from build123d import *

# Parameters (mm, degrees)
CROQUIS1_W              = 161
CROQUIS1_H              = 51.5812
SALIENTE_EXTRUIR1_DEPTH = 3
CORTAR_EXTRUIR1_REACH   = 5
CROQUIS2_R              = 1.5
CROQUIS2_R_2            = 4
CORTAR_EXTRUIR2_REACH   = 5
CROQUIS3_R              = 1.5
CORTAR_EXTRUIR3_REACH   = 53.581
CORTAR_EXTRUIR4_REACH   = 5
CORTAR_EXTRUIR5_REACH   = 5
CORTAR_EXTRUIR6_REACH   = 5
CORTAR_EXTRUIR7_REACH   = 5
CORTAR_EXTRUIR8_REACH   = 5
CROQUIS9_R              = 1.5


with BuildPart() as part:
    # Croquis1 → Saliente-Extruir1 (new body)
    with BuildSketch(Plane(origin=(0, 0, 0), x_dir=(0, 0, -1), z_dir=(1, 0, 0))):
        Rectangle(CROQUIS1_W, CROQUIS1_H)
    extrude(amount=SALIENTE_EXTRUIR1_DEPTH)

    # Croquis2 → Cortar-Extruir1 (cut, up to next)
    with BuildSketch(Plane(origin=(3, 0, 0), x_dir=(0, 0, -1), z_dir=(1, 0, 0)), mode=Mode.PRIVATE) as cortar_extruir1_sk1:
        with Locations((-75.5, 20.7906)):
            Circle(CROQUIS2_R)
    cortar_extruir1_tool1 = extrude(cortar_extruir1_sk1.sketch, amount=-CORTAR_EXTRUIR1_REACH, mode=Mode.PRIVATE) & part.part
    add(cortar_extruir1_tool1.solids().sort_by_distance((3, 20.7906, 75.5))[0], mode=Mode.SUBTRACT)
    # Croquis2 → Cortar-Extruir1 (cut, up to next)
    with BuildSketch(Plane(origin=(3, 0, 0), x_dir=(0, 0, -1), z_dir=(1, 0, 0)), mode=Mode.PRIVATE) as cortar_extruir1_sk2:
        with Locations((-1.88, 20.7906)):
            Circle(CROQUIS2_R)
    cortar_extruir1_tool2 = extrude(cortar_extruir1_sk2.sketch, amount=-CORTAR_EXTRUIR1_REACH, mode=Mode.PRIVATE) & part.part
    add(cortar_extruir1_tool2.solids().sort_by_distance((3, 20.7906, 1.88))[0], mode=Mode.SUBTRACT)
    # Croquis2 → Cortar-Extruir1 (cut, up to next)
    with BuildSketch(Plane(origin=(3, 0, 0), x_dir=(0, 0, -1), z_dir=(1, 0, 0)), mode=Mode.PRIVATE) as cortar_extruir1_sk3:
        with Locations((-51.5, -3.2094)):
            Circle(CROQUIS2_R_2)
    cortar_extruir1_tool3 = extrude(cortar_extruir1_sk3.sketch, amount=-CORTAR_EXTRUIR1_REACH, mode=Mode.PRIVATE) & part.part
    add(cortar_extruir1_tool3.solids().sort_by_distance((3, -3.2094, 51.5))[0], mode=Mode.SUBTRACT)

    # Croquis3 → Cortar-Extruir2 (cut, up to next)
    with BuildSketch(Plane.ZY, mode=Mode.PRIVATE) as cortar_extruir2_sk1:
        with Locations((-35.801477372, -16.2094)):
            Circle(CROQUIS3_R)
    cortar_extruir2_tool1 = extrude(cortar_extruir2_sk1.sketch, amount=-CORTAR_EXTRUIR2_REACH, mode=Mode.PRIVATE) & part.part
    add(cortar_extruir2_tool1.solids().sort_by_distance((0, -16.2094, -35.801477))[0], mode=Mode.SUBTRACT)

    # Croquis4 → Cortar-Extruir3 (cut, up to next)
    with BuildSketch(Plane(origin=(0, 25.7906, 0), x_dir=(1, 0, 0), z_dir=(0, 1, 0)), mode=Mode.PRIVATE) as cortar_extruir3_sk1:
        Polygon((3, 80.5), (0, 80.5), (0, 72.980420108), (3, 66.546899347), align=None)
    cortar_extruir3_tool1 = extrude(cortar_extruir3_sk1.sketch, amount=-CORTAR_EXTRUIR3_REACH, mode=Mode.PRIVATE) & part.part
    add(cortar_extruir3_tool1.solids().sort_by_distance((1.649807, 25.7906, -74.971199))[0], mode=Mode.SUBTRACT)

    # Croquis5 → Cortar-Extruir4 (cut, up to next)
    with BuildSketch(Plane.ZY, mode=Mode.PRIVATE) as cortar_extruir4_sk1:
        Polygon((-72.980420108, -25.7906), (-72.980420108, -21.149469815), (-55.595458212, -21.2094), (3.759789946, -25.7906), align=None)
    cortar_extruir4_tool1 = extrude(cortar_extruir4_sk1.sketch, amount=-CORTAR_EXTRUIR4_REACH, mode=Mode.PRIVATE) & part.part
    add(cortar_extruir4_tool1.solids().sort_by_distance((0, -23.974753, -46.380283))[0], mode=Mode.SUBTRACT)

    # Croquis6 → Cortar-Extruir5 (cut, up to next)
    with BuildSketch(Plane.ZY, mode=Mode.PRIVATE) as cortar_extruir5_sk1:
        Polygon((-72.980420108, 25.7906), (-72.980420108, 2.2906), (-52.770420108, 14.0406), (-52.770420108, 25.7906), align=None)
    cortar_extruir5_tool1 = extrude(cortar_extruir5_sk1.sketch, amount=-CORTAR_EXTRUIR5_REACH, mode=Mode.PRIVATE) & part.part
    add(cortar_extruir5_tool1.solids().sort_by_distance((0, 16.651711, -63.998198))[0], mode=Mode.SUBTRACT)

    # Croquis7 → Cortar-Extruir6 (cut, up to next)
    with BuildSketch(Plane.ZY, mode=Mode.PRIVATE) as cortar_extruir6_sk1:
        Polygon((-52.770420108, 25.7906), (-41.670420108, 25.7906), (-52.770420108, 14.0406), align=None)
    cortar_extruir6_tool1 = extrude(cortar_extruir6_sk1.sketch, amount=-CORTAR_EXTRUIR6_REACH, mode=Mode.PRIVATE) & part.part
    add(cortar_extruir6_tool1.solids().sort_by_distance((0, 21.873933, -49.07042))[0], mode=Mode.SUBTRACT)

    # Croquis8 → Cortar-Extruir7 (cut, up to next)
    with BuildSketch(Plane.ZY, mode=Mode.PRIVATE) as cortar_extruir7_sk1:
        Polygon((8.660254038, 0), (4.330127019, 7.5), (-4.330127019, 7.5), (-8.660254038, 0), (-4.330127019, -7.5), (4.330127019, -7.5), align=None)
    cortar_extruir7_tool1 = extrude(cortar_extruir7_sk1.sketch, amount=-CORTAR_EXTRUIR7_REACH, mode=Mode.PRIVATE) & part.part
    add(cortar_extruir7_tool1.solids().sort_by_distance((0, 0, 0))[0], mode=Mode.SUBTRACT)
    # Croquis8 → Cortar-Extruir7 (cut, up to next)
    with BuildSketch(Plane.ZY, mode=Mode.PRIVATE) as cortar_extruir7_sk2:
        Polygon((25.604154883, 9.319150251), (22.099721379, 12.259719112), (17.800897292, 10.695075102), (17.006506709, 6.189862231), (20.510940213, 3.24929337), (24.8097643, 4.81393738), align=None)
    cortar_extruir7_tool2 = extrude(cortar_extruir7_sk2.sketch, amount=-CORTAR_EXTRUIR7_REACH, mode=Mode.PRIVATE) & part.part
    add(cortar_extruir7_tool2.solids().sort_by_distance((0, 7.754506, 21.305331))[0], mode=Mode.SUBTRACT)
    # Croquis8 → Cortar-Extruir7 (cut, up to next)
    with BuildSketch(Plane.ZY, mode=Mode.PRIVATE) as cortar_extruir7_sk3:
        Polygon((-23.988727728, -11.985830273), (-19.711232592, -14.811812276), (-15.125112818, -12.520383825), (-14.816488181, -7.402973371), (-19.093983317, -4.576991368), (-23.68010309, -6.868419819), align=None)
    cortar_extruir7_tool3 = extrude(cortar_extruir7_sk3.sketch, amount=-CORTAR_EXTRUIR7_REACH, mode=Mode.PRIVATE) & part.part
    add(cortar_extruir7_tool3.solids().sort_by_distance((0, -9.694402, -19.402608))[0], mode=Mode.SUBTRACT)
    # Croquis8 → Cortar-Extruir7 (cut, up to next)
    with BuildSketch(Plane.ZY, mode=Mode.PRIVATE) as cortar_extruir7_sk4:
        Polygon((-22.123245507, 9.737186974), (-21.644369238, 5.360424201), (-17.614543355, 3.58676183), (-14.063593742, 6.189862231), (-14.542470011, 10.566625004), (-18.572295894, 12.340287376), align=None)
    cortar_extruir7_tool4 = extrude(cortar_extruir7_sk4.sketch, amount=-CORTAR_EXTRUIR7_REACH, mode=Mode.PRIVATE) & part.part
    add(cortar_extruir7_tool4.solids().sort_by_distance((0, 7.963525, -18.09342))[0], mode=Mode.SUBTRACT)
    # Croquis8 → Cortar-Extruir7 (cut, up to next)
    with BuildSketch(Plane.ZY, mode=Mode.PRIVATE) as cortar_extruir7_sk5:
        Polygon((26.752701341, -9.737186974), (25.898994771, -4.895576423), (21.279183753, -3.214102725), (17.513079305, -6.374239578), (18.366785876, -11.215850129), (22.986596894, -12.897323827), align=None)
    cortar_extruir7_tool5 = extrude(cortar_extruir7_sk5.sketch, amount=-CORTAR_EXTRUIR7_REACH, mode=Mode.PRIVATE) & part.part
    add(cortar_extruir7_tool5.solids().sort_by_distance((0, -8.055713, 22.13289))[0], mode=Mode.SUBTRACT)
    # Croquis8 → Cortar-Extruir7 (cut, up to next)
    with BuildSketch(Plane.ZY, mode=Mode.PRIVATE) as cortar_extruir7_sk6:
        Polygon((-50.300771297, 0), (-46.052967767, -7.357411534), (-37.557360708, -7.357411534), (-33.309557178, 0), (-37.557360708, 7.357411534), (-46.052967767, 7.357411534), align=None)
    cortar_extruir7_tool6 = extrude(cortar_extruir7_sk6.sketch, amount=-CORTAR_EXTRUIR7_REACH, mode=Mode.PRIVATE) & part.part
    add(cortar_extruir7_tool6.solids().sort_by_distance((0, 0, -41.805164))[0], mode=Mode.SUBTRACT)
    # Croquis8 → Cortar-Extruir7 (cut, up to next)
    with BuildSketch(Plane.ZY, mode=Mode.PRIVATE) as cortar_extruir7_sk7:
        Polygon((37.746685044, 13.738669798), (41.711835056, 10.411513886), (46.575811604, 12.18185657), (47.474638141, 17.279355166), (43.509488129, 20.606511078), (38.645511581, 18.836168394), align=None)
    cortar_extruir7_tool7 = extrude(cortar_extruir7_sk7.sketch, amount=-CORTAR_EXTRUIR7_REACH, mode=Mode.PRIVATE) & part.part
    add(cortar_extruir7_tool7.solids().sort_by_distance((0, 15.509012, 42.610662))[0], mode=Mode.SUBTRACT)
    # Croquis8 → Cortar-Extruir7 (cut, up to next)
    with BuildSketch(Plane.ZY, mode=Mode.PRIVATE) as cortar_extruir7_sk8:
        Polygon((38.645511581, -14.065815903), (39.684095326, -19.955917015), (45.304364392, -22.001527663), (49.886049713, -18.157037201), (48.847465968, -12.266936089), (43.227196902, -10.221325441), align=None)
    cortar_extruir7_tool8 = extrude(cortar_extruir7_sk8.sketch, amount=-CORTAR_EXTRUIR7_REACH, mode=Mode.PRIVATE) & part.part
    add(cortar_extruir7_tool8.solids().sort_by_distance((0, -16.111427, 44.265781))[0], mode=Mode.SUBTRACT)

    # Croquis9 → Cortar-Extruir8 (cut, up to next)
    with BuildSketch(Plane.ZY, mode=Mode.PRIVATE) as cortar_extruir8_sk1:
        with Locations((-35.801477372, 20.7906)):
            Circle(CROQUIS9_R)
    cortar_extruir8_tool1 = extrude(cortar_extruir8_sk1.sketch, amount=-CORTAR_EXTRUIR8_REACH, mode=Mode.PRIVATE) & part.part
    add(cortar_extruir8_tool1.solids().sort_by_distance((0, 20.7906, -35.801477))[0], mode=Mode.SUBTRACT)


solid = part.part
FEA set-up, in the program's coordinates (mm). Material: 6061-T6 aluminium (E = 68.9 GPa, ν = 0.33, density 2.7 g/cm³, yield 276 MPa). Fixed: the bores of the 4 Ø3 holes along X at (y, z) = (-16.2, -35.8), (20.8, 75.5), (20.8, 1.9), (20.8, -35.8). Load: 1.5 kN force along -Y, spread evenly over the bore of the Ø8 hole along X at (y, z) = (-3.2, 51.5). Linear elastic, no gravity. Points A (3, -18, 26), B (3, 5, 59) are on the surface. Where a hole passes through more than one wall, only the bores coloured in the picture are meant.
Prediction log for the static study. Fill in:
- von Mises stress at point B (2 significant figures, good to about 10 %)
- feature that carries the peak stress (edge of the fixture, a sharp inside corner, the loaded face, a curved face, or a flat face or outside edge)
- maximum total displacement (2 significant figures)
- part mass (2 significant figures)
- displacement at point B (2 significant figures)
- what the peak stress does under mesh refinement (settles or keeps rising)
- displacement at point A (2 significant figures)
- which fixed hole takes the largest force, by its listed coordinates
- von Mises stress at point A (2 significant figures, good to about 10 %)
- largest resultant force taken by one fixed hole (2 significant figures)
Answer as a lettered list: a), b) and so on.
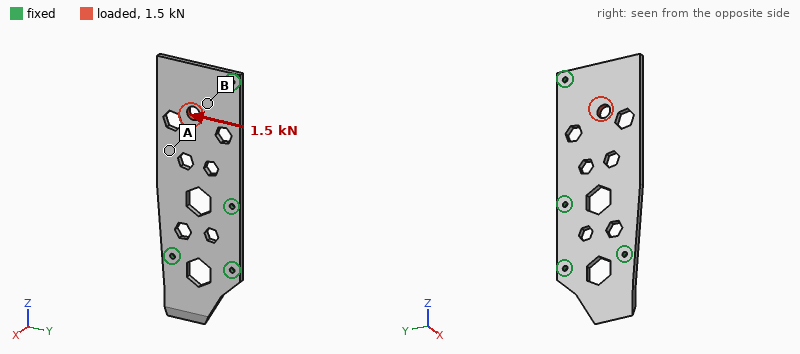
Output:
a) 17 MPa
b) edge of the fixture
c) 17 µm
d) 51 g
e) 12 µm
f) keeps rising
g) 9.9 µm
h) (20.8, 75.5)
i) 7.9 MPa
j) 1.1 kN
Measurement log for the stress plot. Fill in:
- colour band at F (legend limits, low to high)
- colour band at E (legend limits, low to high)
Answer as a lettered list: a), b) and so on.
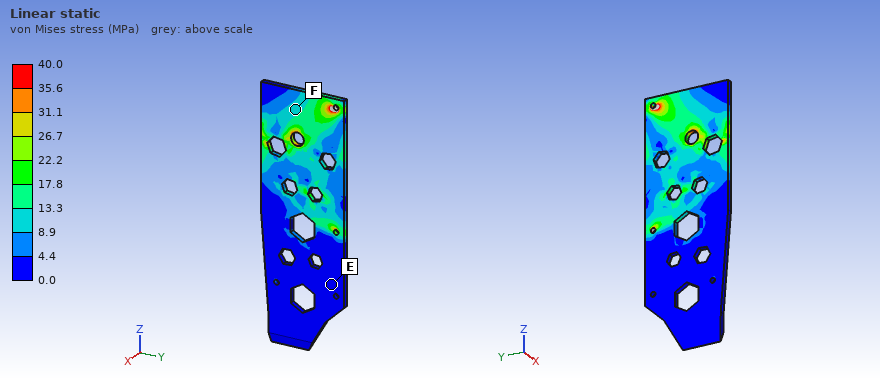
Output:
a) 8.9 to 13.3 MPa
b) 0.0 to 4.4 MPa
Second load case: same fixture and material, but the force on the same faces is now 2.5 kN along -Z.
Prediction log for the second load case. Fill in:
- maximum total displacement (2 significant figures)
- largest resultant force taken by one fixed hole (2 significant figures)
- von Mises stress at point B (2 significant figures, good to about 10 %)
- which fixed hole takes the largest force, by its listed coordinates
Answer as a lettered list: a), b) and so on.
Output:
a) 22 µm
b) 1.1 kN
c) 20 MPa
d) (20.8, 75.5)
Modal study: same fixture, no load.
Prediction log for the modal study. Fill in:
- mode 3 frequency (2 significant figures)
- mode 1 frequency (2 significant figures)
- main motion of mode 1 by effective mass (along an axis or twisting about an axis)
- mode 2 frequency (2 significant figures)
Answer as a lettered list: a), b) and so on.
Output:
a) 2000 Hz
b) 930 Hz
c) along X
d) 2000 Hz
